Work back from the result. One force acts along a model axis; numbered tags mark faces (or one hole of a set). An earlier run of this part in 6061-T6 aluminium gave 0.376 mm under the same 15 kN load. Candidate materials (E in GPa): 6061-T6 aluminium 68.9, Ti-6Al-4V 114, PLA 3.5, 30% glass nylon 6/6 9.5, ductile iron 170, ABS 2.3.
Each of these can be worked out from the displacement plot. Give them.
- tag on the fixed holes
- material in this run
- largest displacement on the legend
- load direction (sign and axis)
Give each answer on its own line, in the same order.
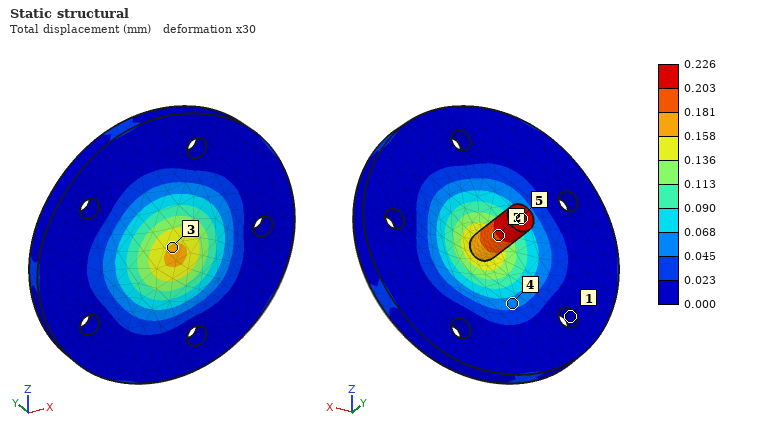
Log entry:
1
Ti-6Al-4V
0.226 mm
-Y
